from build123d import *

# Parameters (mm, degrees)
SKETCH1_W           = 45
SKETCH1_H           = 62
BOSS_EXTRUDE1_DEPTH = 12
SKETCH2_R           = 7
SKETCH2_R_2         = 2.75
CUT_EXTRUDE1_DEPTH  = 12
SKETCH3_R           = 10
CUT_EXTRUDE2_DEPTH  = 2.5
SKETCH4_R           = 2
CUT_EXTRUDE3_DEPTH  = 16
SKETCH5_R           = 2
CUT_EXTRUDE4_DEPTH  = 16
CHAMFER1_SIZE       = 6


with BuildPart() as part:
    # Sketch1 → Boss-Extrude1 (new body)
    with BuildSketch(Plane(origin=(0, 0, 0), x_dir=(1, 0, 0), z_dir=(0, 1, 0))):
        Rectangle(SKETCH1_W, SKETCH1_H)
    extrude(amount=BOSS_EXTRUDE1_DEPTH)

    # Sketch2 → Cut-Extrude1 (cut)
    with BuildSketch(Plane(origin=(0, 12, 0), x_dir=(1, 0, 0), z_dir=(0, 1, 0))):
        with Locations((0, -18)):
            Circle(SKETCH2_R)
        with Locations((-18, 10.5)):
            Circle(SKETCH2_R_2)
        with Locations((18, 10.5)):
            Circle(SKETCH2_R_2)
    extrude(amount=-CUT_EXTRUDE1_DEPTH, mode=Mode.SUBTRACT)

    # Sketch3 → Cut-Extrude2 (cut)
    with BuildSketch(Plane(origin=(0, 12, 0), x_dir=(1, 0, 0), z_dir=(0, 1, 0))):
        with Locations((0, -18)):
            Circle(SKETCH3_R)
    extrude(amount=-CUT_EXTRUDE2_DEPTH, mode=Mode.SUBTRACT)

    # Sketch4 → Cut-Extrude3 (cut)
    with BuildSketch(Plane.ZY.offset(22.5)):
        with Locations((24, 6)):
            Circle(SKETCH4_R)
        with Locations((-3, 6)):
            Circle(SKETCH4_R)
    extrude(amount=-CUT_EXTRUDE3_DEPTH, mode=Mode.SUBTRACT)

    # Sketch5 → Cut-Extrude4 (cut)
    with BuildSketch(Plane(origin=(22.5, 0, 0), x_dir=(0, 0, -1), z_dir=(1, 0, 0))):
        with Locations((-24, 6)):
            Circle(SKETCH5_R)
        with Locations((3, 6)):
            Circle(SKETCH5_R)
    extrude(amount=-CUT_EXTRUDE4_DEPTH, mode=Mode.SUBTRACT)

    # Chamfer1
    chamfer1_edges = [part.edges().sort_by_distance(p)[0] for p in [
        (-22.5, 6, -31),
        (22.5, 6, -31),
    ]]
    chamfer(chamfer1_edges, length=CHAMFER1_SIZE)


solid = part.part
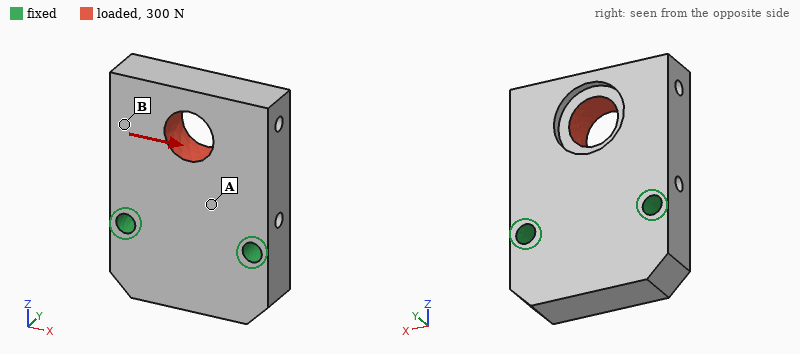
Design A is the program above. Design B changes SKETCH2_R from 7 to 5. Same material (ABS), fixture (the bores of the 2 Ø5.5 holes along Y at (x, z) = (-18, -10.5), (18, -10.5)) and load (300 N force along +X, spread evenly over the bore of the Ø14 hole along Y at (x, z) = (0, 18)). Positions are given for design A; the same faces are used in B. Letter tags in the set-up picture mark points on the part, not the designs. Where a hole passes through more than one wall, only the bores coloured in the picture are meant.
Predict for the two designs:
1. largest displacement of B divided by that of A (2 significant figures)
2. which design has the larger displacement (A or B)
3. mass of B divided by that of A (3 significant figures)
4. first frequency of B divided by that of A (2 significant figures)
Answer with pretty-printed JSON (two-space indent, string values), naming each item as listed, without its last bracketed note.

{
  "largest displacement of B divided by that of A": "0.85",
  "which design has the larger displacement": "A",
  "mass of B divided by that of A": "1.02",
  "first frequency of B divided by that of A": "0.98"
}
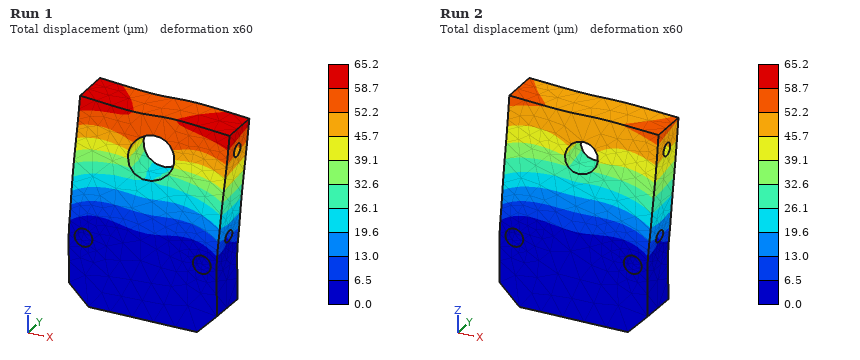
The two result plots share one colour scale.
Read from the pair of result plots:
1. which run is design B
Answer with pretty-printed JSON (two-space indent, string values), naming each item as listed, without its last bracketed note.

{
  "which run is design B": "Run 2"
}
